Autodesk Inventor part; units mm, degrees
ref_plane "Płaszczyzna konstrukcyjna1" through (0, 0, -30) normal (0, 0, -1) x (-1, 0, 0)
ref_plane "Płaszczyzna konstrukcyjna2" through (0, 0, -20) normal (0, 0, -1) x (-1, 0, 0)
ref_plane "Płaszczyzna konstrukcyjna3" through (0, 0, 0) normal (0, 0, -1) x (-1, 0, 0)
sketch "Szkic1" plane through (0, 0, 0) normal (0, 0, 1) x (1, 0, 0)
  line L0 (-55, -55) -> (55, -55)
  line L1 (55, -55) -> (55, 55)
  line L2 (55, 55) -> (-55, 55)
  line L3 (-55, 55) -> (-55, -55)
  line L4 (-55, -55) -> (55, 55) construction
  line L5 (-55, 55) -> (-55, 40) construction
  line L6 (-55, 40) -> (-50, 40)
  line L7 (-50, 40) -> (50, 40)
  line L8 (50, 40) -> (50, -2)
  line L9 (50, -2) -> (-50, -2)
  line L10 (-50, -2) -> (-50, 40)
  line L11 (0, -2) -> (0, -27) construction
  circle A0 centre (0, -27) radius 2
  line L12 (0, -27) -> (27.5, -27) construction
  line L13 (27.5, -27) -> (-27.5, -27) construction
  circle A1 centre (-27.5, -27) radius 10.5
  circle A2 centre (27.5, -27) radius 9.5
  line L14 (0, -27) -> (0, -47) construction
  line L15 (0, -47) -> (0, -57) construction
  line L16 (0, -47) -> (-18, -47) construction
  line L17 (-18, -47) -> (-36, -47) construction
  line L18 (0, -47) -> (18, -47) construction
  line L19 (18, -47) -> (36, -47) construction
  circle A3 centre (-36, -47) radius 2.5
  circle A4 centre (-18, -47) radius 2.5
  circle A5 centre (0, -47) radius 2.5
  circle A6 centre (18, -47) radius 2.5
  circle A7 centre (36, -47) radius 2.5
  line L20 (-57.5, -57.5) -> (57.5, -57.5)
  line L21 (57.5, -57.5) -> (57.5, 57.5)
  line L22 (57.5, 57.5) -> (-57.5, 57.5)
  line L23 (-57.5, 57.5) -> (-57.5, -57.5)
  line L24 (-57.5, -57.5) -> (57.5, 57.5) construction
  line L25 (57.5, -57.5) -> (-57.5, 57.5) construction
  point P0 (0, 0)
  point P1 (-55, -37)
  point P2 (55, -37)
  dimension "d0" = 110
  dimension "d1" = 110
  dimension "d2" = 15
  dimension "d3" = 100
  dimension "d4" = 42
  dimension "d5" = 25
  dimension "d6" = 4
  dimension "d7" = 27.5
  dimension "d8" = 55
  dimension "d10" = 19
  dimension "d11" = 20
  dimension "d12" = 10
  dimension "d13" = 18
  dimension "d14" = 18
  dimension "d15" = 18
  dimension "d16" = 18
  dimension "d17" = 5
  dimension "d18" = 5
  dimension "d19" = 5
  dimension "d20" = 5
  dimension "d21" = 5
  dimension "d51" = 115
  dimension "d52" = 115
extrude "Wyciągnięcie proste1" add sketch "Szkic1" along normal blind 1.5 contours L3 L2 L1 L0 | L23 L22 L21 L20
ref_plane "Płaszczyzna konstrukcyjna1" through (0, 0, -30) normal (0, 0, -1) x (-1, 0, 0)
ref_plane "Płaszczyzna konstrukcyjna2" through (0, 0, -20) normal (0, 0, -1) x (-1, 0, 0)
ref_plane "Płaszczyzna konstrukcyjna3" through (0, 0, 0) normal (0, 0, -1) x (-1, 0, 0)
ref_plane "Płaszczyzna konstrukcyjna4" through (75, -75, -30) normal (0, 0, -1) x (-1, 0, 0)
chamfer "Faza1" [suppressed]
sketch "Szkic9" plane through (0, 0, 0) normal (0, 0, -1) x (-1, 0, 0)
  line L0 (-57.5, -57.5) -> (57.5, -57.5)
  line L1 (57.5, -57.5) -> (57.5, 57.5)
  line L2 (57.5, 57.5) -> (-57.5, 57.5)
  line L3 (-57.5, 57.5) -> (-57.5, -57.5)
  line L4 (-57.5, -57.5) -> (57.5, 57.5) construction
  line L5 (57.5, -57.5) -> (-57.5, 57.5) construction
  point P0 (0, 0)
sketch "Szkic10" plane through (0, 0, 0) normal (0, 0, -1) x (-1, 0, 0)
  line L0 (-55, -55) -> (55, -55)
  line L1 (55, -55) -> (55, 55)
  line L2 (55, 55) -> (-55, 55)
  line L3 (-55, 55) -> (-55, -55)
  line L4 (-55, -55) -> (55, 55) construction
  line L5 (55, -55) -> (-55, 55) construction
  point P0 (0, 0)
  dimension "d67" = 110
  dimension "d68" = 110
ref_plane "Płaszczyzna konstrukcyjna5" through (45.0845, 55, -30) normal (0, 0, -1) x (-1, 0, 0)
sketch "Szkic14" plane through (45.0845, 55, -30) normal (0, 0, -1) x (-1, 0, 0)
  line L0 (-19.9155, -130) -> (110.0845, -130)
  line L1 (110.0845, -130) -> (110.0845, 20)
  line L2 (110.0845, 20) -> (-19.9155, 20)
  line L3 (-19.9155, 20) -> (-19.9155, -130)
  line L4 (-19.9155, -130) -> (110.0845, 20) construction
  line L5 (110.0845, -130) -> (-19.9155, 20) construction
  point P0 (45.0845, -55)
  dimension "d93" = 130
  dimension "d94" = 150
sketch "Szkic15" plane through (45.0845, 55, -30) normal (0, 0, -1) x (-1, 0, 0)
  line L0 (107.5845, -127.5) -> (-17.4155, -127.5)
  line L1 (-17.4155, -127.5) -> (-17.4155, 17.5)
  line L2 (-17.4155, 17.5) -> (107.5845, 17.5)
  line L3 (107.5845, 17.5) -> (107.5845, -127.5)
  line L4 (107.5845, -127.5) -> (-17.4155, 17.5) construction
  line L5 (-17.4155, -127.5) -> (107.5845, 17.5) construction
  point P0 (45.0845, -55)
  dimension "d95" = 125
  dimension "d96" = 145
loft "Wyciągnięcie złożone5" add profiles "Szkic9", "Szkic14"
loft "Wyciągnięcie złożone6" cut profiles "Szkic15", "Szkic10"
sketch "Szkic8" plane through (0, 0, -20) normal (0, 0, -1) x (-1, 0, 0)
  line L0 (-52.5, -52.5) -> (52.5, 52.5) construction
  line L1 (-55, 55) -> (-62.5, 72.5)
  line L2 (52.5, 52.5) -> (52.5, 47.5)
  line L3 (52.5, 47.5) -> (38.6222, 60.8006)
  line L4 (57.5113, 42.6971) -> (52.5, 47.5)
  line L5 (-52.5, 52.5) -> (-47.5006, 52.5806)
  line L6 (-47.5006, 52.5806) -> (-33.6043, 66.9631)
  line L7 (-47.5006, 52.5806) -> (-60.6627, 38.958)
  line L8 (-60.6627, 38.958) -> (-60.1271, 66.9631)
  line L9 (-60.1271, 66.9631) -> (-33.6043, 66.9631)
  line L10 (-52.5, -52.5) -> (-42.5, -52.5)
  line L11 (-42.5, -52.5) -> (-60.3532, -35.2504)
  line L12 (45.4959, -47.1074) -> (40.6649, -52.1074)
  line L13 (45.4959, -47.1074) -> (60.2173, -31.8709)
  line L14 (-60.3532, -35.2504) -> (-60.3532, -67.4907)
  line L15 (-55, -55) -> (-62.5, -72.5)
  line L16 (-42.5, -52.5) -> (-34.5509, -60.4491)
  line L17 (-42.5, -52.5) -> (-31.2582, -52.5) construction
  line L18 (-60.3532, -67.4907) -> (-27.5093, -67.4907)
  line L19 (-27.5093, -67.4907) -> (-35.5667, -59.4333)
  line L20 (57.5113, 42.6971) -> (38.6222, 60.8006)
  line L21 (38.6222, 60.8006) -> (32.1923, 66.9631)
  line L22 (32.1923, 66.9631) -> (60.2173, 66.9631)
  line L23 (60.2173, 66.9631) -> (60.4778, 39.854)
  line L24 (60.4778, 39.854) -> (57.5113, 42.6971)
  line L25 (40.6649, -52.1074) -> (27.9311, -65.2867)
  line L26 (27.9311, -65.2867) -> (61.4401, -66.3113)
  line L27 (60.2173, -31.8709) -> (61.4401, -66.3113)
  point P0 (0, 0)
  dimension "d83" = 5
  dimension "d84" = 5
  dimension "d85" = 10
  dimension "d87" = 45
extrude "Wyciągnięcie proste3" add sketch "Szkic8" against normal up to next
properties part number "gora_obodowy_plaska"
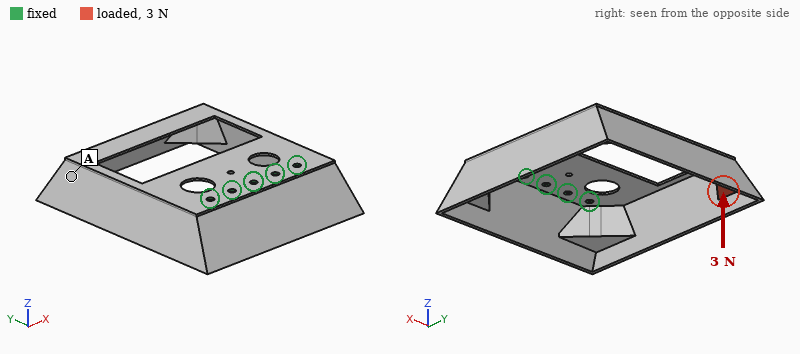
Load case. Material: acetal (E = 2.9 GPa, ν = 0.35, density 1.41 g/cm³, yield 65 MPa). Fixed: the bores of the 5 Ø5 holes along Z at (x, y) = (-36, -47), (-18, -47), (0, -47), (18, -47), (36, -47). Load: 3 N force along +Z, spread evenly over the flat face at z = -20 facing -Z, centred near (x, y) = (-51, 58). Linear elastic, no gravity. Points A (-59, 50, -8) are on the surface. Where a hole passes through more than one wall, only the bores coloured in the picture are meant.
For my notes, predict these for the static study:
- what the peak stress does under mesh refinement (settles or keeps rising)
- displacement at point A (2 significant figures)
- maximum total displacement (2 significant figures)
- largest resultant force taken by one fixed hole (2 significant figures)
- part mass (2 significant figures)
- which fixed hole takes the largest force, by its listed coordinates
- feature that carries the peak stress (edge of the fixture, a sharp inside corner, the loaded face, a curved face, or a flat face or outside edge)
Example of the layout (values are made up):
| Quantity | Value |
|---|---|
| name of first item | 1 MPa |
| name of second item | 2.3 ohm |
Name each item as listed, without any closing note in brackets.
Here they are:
| Quantity | Value |
|---|---|
| what the peak stress does under mesh refinement | keeps rising |
| displacement at point A | 1.7 mm |
| maximum total displacement | 2.2 mm |
| largest resultant force taken by one fixed hole | 10 N |
| part mass | 98 g |
| which fixed hole takes the largest force, by its listed coordinates | (-36, -47) |
| feature that carries the peak stress | edge of the fixture |
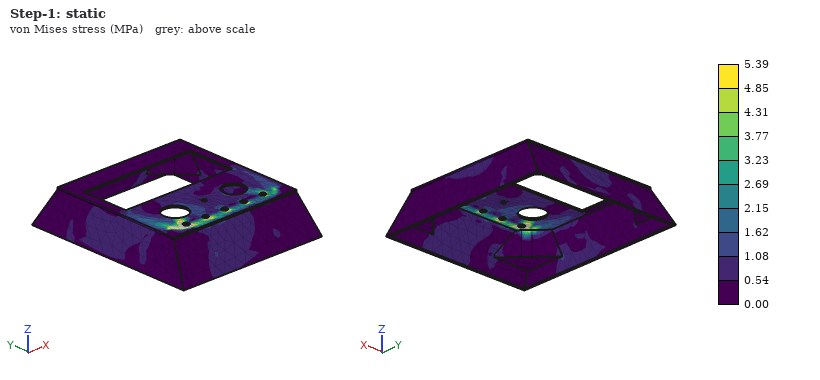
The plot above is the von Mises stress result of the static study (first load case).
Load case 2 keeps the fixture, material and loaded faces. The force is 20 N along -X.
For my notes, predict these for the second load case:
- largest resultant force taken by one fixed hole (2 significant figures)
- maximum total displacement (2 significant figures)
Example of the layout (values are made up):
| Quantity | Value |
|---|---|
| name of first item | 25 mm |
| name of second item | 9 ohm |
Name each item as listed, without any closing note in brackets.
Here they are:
| Quantity | Value |
|---|---|
| largest resultant force taken by one fixed hole | 26 N |
| maximum total displacement | 2.0 mm |
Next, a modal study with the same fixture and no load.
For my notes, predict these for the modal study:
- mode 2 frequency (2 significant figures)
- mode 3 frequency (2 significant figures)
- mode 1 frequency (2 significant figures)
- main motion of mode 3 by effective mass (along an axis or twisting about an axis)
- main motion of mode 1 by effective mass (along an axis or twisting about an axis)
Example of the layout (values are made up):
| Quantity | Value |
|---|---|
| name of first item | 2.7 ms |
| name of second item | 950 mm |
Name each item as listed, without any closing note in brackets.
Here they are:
| Quantity | Value |
|---|---|
| mode 2 frequency | 69 Hz |
| mode 3 frequency | 170 Hz |
| mode 1 frequency | 37 Hz |
| main motion of mode 3 by effective mass | along X |
| main motion of mode 1 by effective mass | along Z |
